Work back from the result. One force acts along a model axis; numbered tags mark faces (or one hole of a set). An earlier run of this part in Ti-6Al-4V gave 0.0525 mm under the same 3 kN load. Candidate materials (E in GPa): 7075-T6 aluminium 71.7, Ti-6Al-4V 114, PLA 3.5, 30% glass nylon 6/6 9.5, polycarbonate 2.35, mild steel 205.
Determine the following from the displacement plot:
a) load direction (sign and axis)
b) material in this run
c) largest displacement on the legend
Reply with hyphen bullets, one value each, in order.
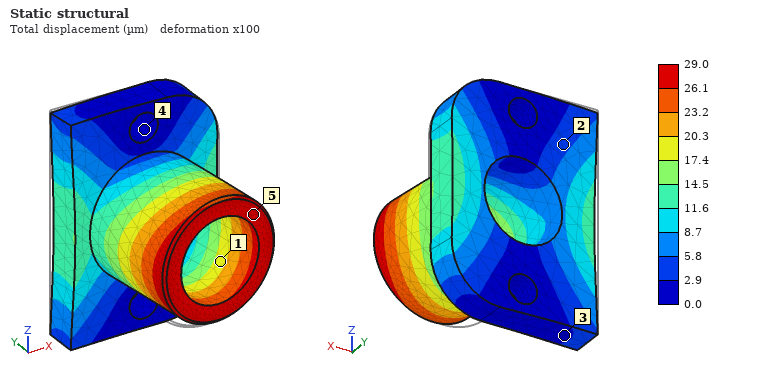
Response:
- +X
- mild steel
- 29.0 µm
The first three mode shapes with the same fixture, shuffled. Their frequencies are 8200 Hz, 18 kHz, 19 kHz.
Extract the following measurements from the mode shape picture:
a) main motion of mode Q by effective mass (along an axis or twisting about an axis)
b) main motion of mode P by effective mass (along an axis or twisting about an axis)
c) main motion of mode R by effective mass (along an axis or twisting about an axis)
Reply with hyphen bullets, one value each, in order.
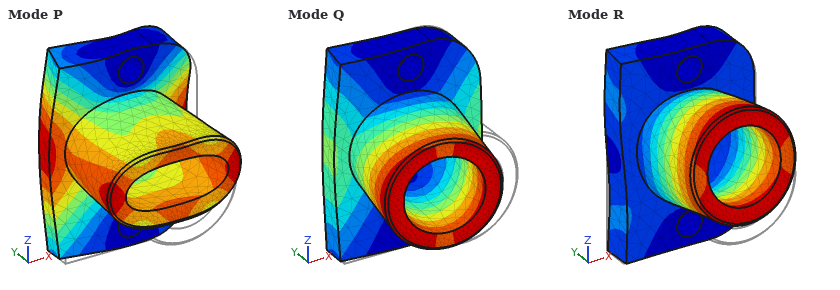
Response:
- along X
- along Y
- along Z
